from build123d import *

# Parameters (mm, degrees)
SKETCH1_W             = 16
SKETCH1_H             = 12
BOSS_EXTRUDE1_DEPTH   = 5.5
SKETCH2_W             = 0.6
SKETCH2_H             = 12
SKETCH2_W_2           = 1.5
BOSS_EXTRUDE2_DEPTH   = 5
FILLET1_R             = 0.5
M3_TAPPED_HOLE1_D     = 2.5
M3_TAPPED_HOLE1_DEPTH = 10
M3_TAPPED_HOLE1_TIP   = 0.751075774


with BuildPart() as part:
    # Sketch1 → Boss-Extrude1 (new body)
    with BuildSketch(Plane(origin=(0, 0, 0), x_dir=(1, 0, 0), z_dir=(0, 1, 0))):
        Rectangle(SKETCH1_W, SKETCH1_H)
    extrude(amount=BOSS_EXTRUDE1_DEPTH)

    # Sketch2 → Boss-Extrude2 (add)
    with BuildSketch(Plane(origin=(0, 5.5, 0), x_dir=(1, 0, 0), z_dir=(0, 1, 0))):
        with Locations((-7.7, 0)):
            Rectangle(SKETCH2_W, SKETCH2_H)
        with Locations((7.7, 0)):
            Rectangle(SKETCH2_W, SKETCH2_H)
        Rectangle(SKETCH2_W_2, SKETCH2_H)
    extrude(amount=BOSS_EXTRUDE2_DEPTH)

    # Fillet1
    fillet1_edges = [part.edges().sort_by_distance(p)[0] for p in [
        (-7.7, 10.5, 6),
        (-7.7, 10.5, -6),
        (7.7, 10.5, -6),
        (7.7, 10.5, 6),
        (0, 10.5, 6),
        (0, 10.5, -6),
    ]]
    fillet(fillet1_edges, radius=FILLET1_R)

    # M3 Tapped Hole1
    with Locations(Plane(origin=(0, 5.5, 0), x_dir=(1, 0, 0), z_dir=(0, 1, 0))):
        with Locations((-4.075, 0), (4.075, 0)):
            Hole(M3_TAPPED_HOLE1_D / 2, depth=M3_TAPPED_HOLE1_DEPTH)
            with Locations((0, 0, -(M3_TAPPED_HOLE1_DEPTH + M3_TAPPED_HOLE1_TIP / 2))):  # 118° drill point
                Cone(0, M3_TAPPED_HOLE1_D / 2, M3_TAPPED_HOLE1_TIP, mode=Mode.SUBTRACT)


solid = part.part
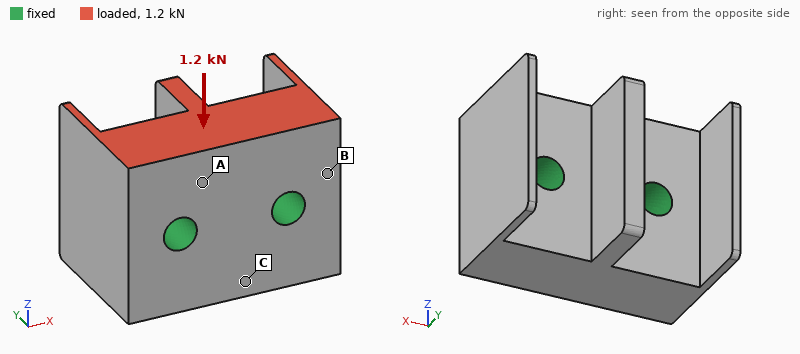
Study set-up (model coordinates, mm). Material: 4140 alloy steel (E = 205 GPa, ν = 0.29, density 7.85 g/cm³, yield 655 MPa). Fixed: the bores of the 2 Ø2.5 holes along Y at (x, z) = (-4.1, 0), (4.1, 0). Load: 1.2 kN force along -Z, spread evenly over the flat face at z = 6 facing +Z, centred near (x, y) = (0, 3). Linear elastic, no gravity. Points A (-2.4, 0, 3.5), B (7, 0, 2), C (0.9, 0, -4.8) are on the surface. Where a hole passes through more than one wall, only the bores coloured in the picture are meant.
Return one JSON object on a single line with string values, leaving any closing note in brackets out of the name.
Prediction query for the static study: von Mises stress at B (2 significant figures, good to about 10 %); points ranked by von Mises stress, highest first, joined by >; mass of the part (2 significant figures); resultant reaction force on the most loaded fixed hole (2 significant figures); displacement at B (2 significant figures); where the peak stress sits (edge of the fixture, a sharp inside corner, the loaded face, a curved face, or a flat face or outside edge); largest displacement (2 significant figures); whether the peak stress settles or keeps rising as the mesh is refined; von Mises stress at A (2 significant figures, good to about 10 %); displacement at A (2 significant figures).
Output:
{"von Mises stress at B": "7.7 MPa", "points ranked by von Mises stress, highest first, joined by >": "A > B > C", "mass of the part": "9.1 g", "resultant reaction force on the most loaded fixed hole": "600 N", "displacement at B": "0.20 µm", "where the peak stress sits": "edge of the fixture", "largest displacement": "0.91 µm", "whether the peak stress settles or keeps rising as the mesh is refined": "keeps rising", "von Mises stress at A": "11 MPa", "displacement at A": "0.16 µm"}
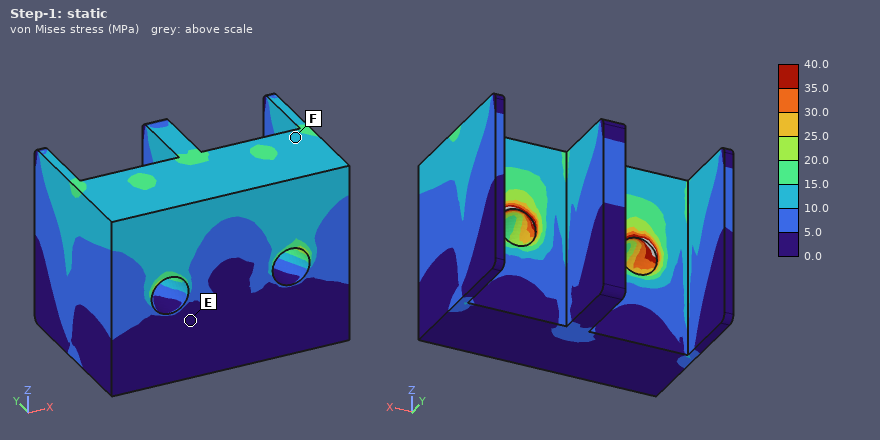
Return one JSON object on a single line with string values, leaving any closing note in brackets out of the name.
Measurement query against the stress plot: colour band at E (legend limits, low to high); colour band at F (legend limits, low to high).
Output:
{"colour band at E": "0.0 to 5.0 MPa", "colour band at F": "10.0 to 15.0 MPa"}
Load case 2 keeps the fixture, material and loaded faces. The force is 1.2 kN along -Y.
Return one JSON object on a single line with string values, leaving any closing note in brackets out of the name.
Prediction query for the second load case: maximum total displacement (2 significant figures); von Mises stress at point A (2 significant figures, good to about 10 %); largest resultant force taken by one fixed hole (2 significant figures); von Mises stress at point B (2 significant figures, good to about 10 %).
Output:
{"maximum total displacement": "3.7 µm", "von Mises stress at point A": "30 MPa", "largest resultant force taken by one fixed hole": "600 N", "von Mises stress at point B": "34 MPa"}
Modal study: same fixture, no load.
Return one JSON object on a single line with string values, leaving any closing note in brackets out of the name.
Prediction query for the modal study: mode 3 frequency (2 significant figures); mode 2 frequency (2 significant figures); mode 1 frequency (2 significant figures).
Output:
{"mode 3 frequency": "25 kHz", "mode 2 frequency": "18 kHz", "mode 1 frequency": "18 kHz"}
